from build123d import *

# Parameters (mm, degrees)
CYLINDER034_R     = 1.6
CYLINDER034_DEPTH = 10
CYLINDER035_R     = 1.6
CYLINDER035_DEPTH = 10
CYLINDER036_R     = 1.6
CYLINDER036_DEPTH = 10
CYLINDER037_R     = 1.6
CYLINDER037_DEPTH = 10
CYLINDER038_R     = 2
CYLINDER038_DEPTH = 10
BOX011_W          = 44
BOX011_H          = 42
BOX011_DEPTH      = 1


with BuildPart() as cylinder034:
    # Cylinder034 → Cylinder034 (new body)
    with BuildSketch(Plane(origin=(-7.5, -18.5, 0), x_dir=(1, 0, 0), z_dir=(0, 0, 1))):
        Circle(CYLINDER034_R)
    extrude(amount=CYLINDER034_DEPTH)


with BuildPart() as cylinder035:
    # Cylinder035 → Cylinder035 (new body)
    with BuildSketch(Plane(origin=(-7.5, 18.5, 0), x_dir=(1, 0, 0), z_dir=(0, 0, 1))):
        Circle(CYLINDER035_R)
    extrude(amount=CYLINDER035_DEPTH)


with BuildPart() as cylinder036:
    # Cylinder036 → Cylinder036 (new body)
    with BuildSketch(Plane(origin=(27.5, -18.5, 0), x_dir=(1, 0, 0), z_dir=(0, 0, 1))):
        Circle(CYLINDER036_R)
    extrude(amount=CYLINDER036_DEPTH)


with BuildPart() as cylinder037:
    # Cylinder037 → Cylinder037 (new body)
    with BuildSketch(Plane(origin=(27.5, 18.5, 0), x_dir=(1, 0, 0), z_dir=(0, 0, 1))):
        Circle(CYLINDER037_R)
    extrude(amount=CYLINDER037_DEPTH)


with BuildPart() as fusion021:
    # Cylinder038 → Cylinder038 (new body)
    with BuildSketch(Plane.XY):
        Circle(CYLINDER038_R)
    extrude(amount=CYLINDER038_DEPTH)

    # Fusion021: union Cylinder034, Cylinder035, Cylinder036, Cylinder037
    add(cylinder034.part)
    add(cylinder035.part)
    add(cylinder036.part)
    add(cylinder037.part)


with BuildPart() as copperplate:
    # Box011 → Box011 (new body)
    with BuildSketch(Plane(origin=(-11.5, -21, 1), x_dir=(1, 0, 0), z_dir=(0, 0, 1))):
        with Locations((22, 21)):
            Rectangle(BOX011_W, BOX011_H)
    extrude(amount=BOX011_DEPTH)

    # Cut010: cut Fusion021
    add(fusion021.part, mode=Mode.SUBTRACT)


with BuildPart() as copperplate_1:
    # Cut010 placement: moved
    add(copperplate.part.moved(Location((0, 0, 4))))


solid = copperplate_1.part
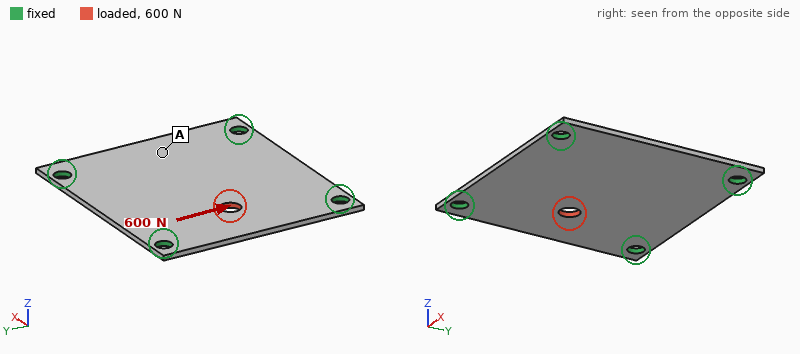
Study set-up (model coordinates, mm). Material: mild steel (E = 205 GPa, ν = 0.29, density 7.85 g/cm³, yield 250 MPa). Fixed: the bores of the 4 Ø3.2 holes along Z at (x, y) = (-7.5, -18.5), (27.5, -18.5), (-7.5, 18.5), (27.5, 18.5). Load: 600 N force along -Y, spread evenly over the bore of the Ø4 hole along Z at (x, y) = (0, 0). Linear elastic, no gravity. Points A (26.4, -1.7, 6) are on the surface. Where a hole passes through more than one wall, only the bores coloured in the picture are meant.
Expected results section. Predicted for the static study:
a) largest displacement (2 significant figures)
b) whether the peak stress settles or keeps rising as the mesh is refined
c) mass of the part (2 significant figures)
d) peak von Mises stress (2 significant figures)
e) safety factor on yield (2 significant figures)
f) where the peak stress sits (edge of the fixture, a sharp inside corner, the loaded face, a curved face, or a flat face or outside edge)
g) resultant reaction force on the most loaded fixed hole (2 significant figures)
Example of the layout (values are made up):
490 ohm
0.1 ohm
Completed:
2.7 µm
settles
14 g
83 MPa
3.0
the loaded face
230 N
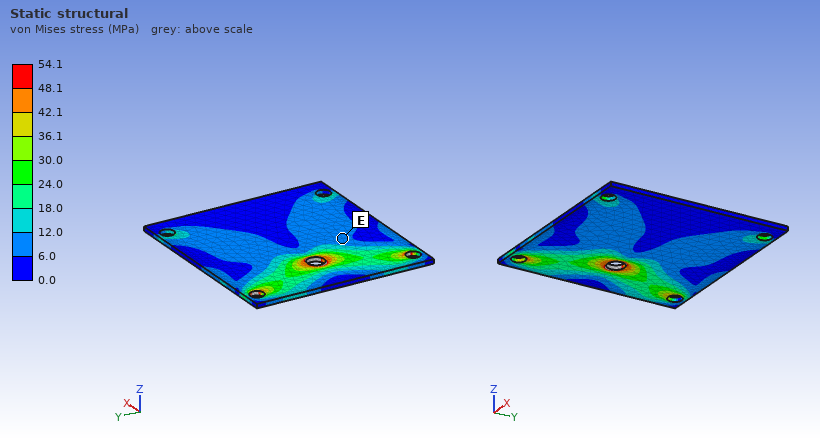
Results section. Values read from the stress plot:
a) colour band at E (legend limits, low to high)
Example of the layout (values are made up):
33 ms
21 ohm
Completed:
6.0 to 12.0 MPa
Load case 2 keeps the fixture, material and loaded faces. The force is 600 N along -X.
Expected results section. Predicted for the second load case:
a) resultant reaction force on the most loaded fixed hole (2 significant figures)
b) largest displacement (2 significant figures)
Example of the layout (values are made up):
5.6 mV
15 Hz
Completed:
180 N
3.8 µm
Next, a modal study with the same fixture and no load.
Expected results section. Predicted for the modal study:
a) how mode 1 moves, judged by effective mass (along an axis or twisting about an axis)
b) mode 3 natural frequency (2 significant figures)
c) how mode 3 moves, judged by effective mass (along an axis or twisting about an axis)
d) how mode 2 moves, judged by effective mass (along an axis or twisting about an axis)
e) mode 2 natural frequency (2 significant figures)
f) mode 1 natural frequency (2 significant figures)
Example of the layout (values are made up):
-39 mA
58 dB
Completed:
along Z
5200 Hz
twisting about X
twisting about Y
4700 Hz
2900 Hz
